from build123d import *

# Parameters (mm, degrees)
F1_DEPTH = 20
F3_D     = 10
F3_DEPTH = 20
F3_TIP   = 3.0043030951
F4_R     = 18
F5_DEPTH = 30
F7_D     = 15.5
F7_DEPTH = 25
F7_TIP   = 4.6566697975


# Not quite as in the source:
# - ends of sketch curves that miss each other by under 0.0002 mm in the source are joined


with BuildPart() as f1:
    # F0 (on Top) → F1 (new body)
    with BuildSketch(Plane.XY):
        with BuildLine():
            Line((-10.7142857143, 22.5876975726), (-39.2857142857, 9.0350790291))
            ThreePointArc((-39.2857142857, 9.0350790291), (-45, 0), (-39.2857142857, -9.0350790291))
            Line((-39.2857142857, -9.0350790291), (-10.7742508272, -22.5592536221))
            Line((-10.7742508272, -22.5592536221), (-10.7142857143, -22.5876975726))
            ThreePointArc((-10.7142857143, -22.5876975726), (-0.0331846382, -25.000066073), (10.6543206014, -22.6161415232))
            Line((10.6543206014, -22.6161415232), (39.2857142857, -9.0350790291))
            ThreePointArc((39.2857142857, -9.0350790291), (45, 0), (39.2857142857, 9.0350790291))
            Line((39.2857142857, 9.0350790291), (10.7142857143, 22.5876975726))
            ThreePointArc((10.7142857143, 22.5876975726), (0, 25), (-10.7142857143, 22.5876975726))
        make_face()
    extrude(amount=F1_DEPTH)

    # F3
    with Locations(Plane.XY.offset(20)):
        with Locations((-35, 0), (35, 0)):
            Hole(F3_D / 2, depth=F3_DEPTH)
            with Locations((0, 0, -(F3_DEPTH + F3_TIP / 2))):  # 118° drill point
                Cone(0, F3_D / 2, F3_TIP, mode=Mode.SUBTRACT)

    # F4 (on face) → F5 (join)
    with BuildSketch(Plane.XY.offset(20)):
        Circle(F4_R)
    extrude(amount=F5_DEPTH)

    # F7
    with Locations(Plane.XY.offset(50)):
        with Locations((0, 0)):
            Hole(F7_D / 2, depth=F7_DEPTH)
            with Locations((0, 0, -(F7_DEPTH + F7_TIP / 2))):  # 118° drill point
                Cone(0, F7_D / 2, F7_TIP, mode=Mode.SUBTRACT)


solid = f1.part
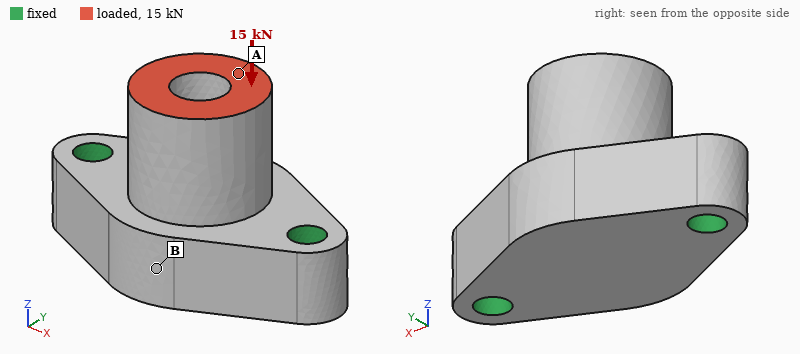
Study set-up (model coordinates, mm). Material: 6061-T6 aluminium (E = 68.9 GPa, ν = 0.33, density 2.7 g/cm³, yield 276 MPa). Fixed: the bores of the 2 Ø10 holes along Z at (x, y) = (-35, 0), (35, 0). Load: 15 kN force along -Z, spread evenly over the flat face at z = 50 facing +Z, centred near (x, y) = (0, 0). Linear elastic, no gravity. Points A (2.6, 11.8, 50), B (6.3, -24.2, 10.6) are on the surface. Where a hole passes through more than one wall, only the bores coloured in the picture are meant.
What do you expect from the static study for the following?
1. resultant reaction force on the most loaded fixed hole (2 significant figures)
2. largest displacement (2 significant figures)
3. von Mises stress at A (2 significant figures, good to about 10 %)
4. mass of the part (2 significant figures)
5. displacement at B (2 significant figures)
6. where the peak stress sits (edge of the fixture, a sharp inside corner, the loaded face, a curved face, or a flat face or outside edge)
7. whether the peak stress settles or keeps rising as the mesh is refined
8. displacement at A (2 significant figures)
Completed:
7.6 kN
26 µm
18 MPa
220 g
20 µm
edge of the fixture
keeps rising
26 µm
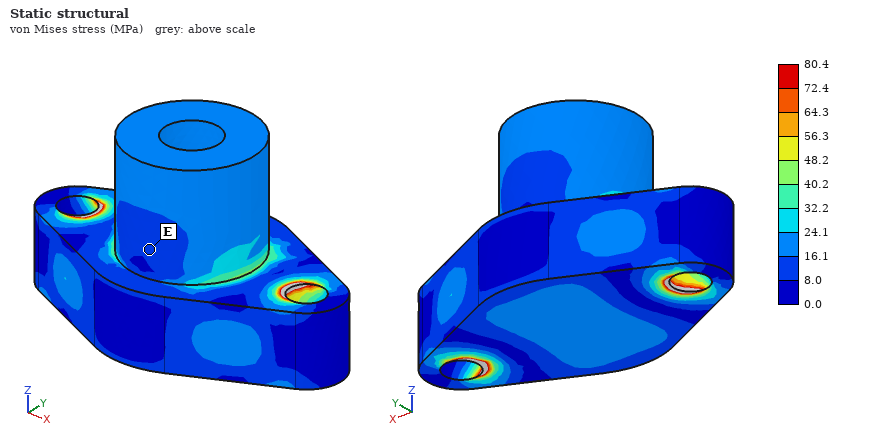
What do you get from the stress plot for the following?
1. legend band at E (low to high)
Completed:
8.0 to 16.1 MPa
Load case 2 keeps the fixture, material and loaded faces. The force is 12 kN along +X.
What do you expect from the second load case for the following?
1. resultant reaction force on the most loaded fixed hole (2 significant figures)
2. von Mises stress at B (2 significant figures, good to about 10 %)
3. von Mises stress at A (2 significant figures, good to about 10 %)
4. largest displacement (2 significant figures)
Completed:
10 kN
12 MPa
34 MPa
93 µm
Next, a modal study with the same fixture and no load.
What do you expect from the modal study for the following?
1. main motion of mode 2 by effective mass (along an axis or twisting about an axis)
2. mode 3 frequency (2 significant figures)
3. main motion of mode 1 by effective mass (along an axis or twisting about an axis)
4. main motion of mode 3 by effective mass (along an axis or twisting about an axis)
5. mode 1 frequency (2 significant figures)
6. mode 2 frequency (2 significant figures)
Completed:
along Z
12 kHz
along Y
along X
6100 Hz
11 kHz
